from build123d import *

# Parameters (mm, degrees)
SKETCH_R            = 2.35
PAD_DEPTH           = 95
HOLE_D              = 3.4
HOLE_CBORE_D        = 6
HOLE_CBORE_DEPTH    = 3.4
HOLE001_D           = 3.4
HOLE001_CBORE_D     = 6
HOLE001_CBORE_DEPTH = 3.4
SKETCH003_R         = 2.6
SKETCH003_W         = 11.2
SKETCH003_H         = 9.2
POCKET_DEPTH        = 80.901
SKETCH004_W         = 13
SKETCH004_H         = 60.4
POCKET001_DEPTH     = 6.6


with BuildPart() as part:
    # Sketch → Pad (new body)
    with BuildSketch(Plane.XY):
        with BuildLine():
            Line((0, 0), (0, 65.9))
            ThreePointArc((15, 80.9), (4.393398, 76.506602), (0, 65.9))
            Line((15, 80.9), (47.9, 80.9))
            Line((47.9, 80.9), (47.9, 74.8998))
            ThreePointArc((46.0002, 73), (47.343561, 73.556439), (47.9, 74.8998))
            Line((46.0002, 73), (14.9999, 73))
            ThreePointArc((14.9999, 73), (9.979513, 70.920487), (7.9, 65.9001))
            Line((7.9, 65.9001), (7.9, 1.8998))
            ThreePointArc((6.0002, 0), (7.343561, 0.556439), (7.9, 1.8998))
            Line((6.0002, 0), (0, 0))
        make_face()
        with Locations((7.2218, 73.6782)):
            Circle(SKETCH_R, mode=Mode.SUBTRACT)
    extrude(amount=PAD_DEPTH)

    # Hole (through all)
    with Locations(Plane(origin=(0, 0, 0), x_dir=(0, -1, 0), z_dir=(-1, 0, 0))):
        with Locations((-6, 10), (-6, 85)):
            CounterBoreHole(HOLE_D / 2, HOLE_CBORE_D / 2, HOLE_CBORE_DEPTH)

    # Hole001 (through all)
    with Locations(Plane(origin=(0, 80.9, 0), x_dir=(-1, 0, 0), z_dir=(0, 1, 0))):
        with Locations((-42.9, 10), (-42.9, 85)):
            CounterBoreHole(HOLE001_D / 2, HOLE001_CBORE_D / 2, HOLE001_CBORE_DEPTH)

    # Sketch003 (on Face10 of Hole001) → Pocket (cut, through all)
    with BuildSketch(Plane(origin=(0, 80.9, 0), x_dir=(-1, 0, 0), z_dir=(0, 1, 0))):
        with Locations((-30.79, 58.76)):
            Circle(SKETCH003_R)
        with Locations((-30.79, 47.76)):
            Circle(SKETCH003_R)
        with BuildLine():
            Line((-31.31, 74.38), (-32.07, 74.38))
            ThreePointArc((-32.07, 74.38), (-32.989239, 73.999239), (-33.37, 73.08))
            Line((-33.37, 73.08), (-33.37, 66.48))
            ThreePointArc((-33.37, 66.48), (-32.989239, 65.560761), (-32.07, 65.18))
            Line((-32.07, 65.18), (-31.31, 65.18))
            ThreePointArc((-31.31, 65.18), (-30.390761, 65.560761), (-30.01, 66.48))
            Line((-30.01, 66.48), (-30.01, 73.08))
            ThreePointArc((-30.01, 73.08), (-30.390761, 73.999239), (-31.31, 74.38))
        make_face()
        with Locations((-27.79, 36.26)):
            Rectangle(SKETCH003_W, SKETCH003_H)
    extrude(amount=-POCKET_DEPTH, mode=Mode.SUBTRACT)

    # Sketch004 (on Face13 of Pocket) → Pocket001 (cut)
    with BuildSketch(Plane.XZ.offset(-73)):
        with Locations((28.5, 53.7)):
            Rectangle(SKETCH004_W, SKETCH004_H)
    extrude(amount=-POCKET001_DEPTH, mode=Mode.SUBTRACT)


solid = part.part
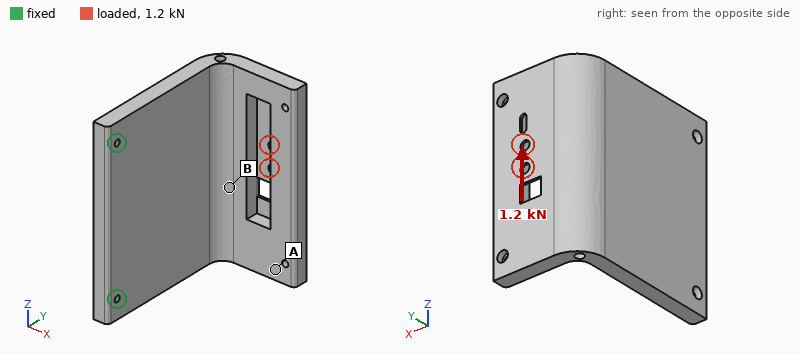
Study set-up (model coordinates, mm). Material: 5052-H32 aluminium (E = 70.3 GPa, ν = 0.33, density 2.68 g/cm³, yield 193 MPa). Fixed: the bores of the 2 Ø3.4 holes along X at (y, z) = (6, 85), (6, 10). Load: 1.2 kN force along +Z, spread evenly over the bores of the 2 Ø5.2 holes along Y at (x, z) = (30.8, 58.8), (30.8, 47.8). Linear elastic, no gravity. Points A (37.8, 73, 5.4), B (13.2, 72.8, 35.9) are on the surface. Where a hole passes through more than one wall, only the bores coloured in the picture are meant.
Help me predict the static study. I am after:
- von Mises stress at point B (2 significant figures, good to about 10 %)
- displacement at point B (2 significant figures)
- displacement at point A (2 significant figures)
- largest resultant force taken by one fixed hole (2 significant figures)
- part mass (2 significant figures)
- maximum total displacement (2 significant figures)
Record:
23 MPa
0.069 mm
0.23 mm
1.4 kN
210 g
0.28 mm
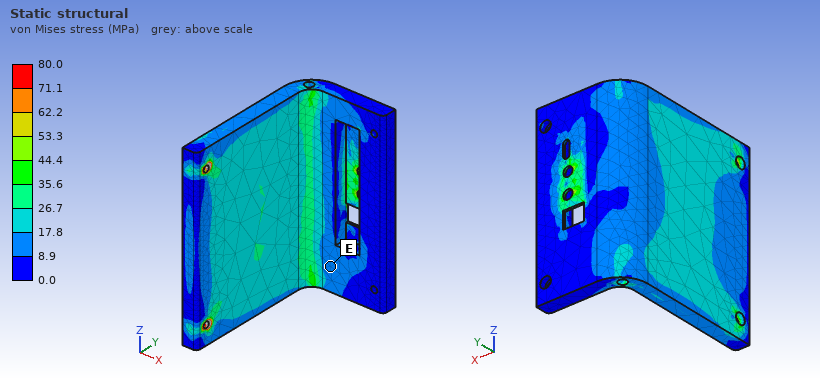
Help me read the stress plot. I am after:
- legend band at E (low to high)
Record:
8.9 to 17.8 MPa
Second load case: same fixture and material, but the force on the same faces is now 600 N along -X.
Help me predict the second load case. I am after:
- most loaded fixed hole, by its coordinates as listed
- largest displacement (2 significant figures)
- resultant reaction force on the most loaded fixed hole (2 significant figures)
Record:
(6, 85)
0.97 mm
360 N
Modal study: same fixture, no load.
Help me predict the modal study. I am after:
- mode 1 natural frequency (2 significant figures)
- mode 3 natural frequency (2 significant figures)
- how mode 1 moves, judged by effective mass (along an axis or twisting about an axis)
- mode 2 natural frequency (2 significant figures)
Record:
440 Hz
1900 Hz
along X
1200 Hz
